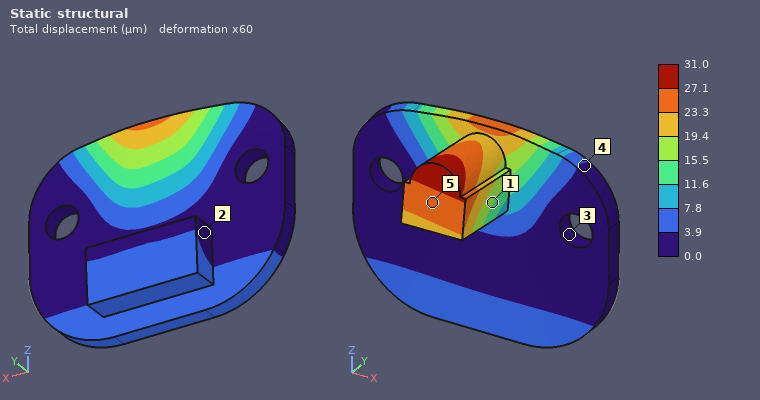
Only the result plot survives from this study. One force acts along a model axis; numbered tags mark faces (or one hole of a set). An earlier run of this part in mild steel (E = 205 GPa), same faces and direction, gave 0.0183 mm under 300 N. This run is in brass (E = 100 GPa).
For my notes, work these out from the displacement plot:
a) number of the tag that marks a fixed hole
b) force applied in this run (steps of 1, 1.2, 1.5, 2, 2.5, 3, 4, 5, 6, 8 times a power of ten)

3
250 N
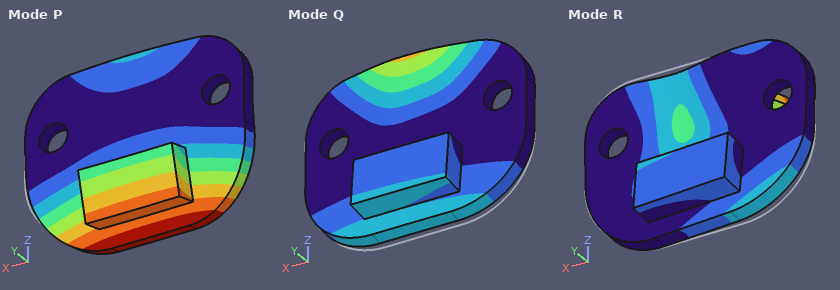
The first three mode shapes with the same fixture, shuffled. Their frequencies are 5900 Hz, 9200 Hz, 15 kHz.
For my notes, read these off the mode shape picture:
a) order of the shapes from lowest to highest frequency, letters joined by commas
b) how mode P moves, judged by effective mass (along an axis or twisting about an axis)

P, Q, R
along Y
